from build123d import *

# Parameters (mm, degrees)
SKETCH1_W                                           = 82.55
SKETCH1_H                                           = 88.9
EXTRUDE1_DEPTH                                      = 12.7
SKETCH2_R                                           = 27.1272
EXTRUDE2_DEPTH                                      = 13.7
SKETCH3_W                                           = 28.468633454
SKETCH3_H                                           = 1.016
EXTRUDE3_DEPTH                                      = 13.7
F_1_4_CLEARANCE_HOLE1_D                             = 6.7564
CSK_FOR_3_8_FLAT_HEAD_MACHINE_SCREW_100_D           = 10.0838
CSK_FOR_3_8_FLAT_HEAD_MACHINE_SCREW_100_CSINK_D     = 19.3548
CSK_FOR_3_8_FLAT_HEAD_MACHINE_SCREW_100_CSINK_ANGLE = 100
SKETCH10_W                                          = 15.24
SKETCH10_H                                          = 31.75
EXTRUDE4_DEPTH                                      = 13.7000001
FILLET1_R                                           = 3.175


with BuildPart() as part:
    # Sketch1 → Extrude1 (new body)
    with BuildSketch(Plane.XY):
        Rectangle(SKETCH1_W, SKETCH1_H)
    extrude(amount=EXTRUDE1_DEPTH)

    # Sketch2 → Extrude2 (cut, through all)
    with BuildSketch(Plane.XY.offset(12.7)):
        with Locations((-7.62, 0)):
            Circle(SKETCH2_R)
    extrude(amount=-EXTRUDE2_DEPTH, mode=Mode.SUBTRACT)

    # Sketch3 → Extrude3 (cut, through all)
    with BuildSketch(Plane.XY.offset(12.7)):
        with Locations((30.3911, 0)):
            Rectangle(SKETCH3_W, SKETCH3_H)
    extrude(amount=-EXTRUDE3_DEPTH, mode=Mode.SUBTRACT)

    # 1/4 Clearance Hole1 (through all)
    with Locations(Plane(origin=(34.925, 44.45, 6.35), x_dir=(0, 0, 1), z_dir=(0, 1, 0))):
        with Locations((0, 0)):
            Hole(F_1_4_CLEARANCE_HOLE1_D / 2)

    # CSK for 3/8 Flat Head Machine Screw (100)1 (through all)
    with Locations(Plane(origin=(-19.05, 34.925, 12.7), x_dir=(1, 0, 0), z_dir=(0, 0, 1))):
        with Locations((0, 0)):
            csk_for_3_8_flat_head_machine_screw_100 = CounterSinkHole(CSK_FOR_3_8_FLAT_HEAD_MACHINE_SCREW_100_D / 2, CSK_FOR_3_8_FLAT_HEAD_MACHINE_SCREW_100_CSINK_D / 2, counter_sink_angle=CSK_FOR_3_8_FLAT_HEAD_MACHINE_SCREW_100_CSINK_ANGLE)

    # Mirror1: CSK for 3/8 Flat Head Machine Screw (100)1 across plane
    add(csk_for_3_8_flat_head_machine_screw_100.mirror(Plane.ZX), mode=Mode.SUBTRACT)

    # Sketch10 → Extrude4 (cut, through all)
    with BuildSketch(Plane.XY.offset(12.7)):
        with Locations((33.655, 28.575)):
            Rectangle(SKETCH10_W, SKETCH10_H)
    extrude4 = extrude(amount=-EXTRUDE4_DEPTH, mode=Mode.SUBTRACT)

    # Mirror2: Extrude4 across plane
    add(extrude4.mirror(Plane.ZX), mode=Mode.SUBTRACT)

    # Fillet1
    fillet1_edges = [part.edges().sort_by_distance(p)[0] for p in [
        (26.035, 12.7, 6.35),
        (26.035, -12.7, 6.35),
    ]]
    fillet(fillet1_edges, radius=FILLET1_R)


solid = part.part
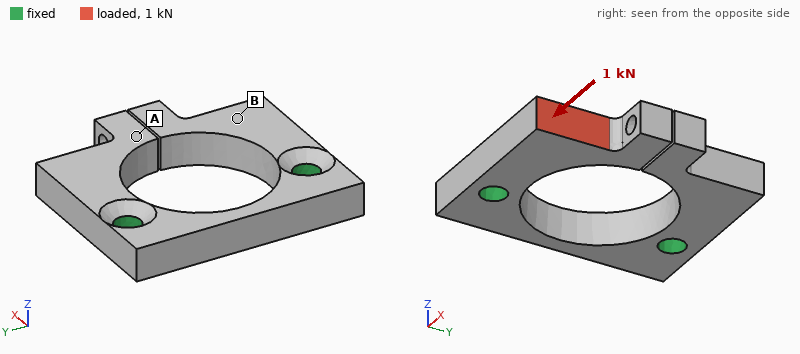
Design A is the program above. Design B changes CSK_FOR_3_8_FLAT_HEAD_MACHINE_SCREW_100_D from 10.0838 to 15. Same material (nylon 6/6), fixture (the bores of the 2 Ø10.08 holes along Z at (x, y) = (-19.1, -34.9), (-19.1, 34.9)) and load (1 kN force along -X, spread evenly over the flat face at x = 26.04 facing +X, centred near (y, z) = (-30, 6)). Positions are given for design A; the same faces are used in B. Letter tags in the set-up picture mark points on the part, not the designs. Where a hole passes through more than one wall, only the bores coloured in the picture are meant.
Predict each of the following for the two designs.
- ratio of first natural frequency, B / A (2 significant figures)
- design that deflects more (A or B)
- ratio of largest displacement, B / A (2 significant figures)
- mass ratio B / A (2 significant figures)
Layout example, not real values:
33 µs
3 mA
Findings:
1.2
A
0.78
0.96
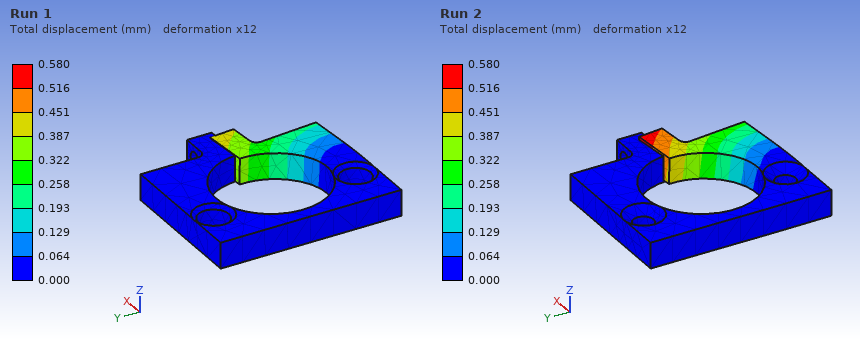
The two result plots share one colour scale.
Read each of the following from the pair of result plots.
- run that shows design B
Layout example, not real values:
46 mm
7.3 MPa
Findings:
Run 1
